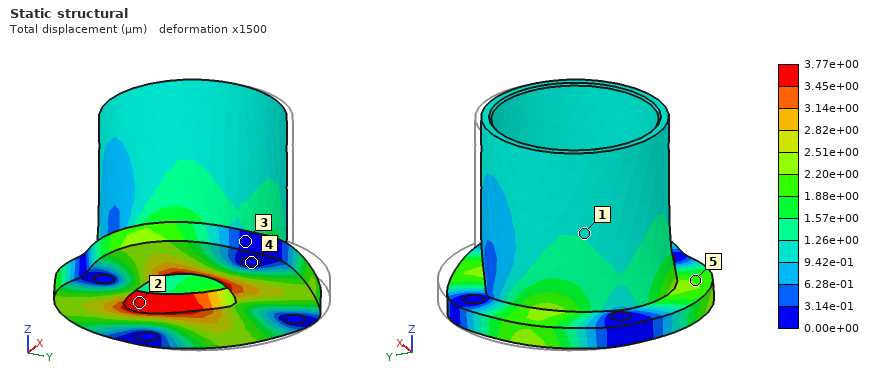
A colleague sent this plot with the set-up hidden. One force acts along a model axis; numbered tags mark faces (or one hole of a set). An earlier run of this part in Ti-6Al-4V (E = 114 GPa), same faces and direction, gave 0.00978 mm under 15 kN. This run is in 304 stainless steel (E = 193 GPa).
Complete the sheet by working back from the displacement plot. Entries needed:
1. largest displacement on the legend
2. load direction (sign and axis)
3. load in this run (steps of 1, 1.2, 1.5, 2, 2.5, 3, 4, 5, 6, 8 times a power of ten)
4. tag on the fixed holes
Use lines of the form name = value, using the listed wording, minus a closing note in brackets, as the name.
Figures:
largest displacement on the legend = 3.77e+00 µm
load direction = -Y
load in this run = 10 kN
tag on the fixed holes = 4
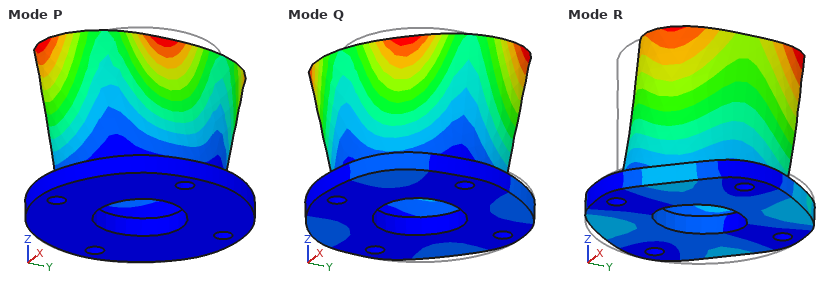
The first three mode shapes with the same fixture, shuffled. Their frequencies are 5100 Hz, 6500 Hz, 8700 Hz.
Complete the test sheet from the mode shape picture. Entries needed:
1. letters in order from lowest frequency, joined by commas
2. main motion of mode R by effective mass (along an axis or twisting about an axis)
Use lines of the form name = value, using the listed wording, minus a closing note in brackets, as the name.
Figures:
letters in order from lowest frequency, joined by commas = Q, P, R
main motion of mode R by effective mass = along X
